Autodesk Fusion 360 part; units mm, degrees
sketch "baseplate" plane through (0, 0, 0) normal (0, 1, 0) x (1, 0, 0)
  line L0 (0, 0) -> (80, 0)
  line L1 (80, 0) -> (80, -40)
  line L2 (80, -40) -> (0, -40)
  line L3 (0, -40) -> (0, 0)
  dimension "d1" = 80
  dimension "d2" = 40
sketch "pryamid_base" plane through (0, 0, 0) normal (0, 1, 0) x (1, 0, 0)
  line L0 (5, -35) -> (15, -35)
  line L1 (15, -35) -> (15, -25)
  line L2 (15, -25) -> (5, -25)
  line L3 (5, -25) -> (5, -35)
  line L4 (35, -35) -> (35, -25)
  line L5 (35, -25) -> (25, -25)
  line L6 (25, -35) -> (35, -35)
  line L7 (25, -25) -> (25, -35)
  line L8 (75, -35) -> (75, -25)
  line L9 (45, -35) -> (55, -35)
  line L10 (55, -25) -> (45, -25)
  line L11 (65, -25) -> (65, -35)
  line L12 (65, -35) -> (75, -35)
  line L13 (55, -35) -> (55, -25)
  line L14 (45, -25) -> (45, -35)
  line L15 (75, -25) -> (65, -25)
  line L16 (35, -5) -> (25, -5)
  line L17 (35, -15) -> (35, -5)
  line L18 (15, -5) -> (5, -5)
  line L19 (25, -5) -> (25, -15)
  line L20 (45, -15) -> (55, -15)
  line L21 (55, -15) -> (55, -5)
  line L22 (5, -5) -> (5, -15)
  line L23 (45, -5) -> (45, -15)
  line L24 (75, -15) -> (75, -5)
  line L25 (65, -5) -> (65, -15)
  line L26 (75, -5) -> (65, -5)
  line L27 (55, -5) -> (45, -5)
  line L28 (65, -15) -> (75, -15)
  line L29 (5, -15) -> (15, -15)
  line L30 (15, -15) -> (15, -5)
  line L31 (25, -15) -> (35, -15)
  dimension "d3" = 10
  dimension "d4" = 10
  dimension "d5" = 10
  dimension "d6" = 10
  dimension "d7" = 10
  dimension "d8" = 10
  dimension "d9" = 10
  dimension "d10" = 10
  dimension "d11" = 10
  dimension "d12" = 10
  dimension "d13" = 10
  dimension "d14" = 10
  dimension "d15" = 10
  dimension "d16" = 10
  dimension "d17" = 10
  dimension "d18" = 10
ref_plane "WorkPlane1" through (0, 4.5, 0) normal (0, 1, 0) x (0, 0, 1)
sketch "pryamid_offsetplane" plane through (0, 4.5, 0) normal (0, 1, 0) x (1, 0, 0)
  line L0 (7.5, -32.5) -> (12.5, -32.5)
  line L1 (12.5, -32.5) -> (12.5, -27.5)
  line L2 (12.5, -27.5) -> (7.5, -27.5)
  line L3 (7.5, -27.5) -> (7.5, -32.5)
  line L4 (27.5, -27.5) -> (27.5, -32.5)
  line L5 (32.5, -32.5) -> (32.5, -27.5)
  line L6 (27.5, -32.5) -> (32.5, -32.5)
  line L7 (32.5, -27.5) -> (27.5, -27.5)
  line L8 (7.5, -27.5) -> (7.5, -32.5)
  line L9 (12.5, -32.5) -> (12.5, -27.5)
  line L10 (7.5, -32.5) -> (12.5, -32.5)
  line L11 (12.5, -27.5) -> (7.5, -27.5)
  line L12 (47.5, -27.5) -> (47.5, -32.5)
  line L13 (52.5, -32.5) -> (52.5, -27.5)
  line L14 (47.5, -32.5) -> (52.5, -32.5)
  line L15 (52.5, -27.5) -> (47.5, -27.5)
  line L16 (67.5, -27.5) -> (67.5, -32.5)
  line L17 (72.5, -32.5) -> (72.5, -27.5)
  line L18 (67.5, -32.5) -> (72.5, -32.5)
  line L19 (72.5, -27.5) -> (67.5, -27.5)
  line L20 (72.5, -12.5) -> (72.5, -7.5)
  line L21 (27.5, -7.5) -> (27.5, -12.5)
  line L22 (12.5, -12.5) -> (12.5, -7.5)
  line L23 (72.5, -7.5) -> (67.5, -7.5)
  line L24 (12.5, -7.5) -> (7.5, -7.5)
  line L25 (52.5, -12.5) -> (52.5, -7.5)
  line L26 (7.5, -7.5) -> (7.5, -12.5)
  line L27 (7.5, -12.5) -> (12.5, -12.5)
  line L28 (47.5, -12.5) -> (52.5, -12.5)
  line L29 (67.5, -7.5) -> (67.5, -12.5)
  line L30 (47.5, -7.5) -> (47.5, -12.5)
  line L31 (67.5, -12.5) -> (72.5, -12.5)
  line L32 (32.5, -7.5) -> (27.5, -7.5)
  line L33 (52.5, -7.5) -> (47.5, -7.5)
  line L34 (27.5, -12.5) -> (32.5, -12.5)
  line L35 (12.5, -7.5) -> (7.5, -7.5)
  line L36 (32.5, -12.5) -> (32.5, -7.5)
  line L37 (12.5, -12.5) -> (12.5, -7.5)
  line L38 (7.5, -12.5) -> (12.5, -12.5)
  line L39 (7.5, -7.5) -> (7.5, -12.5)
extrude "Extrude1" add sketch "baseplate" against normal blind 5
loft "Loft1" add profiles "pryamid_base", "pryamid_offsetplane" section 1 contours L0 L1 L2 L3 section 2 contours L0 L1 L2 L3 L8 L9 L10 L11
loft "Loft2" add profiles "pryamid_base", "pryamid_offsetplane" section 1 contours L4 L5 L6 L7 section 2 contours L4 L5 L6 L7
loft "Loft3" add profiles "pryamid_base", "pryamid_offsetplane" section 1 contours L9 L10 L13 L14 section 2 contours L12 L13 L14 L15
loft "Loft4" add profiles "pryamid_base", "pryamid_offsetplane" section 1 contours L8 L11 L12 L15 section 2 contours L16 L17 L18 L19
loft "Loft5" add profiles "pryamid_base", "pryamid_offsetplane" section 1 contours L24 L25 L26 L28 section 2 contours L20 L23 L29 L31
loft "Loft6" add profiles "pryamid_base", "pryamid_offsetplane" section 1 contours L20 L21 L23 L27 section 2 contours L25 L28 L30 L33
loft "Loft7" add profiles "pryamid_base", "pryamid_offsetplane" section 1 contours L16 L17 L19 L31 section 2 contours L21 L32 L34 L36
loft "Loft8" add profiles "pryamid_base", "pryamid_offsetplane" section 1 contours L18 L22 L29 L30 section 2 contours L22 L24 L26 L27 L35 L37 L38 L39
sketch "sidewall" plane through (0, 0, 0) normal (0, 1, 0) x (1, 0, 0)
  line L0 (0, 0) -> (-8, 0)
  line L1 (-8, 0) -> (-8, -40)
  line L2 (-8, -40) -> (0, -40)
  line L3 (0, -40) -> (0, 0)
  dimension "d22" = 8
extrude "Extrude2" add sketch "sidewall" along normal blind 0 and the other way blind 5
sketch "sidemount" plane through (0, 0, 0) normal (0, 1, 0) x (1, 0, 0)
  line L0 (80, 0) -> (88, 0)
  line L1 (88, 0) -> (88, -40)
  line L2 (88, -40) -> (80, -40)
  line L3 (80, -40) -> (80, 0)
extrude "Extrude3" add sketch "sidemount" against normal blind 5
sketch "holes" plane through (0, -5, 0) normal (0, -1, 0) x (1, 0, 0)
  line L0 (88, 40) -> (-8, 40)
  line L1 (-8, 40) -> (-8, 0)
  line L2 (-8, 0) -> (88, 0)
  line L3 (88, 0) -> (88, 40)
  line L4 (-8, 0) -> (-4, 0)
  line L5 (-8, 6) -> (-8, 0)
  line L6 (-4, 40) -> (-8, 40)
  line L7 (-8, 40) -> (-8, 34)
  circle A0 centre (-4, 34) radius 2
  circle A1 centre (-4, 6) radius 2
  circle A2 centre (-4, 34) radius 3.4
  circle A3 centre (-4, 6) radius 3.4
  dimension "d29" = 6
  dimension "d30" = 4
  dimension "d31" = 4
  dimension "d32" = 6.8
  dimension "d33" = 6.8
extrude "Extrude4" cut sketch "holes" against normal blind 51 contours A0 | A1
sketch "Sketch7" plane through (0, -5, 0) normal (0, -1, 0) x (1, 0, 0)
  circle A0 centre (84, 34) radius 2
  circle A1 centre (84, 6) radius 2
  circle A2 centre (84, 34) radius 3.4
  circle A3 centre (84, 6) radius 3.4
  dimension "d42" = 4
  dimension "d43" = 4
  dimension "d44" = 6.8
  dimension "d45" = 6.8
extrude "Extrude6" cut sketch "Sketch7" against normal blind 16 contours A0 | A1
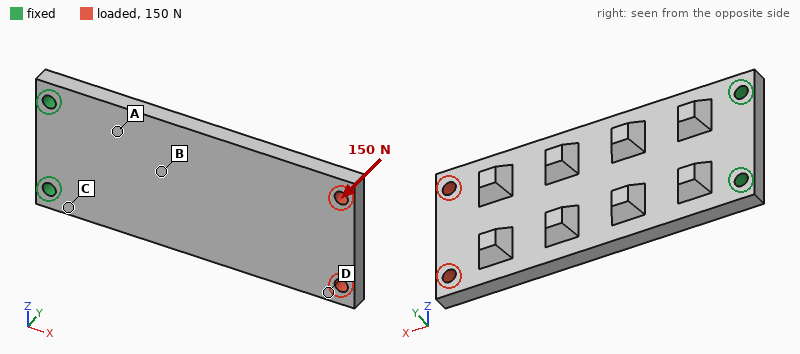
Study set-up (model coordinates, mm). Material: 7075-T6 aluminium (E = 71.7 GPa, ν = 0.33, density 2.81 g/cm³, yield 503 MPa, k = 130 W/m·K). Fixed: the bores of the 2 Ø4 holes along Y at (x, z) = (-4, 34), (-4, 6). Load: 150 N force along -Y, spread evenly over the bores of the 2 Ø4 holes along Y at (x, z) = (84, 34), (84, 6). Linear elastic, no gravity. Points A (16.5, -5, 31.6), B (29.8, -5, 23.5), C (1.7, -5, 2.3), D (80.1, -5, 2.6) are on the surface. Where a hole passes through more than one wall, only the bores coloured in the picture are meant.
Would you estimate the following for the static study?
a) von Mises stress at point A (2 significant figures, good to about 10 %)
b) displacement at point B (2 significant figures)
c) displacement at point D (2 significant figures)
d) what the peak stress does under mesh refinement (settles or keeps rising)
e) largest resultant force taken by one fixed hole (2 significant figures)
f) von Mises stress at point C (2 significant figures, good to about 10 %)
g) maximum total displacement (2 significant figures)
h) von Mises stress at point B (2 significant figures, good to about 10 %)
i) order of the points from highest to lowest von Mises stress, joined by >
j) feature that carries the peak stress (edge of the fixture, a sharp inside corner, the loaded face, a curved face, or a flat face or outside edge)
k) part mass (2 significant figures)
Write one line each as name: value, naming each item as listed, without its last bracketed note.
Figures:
von Mises stress at point A: 57 MPa
displacement at point B: 0.22 mm
displacement at point D: 0.97 mm
what the peak stress does under mesh refinement: keeps rising
largest resultant force taken by one fixed hole: 75 N
von Mises stress at point C: 82 MPa
maximum total displacement: 1.1 mm
von Mises stress at point B: 35 MPa
order of the points from highest to lowest von Mises stress, joined by >: C > A > B > D
feature that carries the peak stress: edge of the fixture
part mass: 59 g
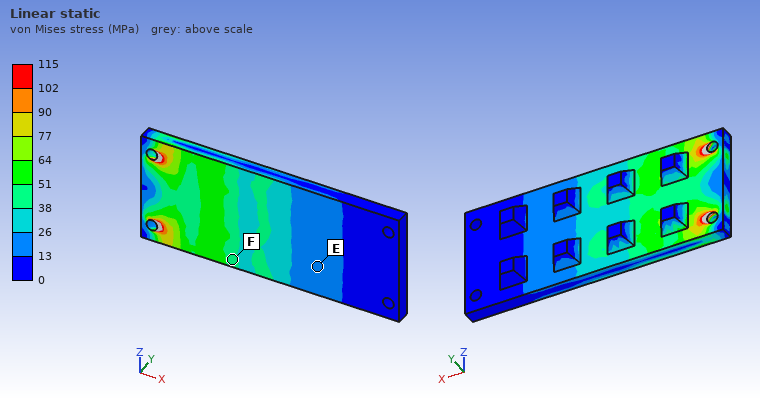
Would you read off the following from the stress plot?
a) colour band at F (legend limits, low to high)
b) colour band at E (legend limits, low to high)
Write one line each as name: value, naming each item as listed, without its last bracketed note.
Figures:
colour band at F: 38 to 51 MPa
colour band at E: 13 to 26 MPa
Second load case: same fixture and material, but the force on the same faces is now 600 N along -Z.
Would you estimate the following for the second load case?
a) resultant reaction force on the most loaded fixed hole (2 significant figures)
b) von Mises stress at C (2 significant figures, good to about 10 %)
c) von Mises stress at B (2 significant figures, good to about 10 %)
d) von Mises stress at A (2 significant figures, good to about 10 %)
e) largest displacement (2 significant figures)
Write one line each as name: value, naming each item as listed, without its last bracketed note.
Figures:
resultant reaction force on the most loaded fixed hole: 1.8 kN
von Mises stress at C: 28 MPa
von Mises stress at B: 9.3 MPa
von Mises stress at A: 18 MPa
largest displacement: 94 µm
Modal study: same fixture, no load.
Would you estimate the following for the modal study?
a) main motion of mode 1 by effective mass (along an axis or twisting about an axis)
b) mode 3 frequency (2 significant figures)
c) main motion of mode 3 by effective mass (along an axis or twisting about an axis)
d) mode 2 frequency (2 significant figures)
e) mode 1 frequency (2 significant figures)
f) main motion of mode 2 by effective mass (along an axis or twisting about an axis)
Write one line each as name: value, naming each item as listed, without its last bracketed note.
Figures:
main motion of mode 1 by effective mass: along Y
mode 3 frequency: 3000 Hz
main motion of mode 3 by effective mass: along Y
mode 2 frequency: 2500 Hz
mode 1 frequency: 480 Hz
main motion of mode 2 by effective mass: twisting about X
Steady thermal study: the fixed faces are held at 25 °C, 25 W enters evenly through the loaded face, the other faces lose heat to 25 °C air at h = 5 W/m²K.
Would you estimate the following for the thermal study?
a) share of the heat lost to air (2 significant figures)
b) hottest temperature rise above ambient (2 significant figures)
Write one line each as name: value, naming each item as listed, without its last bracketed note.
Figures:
share of the heat lost to air: 7.6 %
hottest temperature rise above ambient: 84 K
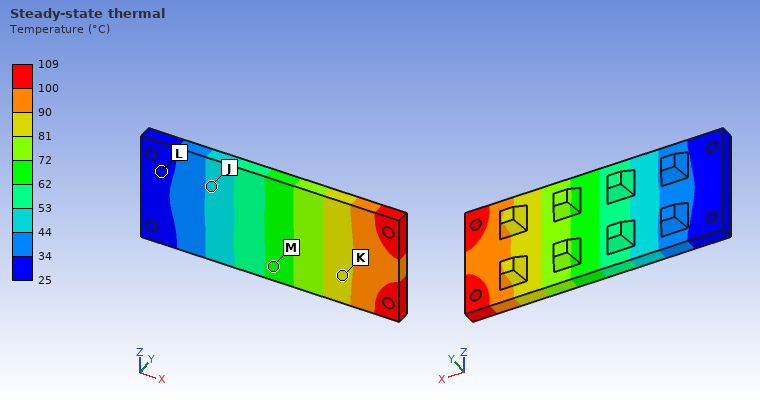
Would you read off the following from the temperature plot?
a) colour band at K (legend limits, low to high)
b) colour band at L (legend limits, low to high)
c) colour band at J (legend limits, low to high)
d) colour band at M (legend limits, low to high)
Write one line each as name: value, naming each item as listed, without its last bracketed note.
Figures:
colour band at K: 81 to 90 °C
colour band at L: 25 to 34 °C
colour band at J: 44 to 53 °C
colour band at M: 62 to 72 °C
